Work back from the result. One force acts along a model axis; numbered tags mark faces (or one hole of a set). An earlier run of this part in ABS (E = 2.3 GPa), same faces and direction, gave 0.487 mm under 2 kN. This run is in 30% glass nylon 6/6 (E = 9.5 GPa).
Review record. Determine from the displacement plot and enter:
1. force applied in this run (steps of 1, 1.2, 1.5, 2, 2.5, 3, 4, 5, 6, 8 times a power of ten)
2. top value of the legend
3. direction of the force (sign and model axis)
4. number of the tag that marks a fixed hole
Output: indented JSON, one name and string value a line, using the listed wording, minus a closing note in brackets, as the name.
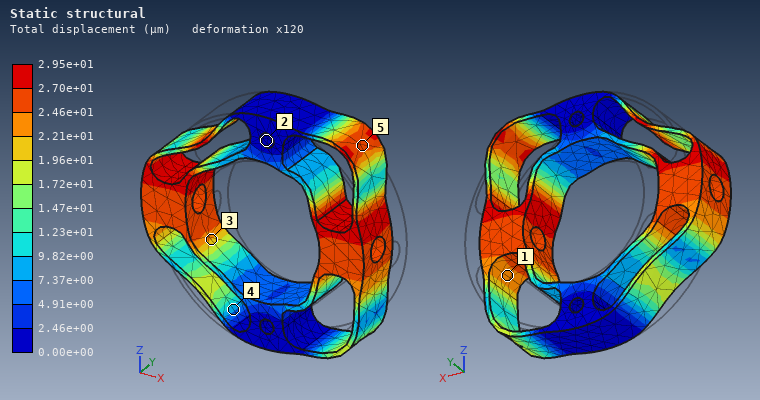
{
  "force applied in this run": "500 N",
  "top value of the legend": "2.95e+01 µm",
  "direction of the force": "-X",
  "number of the tag that marks a fixed hole": "2"
}
